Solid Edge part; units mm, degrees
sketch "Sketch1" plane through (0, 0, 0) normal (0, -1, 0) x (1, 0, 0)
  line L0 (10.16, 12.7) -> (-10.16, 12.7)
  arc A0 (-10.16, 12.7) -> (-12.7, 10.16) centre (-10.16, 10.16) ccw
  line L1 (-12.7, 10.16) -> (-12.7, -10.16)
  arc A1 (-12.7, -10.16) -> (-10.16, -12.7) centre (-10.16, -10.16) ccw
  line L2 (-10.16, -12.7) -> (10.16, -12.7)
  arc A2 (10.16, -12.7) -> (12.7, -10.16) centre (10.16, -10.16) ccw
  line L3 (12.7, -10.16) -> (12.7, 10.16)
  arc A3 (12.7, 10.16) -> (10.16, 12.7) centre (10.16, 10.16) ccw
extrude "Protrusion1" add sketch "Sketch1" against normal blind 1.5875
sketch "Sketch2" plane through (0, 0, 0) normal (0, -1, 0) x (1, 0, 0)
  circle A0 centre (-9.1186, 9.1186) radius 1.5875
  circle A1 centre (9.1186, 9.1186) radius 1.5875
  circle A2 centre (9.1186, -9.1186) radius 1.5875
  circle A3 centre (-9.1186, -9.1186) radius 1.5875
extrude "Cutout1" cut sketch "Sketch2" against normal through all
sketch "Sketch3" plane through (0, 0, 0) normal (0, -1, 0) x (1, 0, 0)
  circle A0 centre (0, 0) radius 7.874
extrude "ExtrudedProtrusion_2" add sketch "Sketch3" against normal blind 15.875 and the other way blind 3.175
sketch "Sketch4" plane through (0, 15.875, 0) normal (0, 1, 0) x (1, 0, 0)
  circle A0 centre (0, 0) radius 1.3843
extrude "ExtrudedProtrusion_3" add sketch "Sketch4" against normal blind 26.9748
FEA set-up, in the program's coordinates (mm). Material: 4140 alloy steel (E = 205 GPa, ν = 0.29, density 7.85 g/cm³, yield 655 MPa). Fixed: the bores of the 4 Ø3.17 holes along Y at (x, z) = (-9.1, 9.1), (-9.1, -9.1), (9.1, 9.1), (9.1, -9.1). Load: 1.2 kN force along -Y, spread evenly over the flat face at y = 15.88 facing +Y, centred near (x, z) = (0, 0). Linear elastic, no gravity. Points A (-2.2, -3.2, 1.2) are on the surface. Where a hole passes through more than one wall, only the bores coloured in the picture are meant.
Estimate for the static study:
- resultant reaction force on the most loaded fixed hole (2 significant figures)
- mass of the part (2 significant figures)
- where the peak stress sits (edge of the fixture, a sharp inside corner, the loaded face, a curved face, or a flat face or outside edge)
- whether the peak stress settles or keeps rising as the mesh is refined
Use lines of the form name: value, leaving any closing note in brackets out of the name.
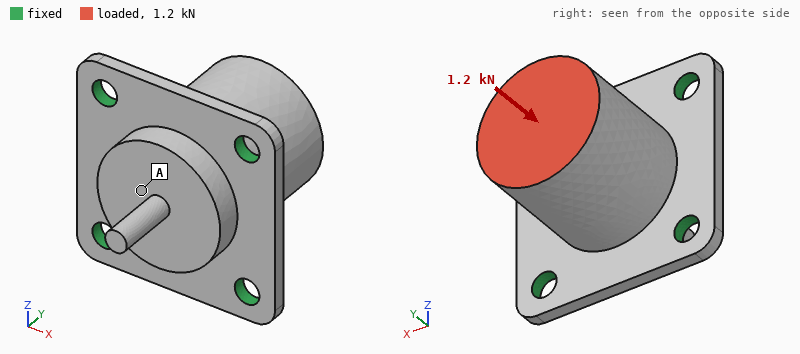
resultant reaction force on the most loaded fixed hole: 300 N
mass of the part: 35 g
where the peak stress sits: edge of the fixture
whether the peak stress settles or keeps rising as the mesh is refined: keeps rising
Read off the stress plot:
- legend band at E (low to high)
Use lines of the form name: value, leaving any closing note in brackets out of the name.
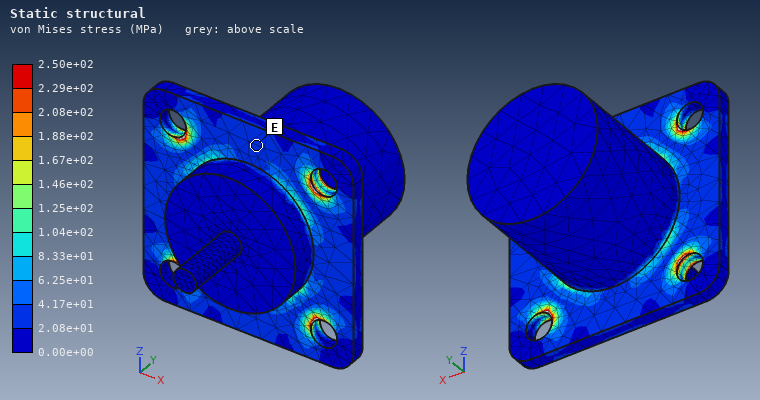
legend band at E: 2.08e+01 to 4.17e+01 MPa
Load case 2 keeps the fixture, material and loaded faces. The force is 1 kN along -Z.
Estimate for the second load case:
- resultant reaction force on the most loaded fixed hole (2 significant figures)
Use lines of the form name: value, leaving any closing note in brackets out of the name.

resultant reaction force on the most loaded fixed hole: 560 N
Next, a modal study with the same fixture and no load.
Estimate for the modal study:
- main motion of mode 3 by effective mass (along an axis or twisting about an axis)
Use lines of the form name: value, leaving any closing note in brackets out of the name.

main motion of mode 3 by effective mass: along Y
